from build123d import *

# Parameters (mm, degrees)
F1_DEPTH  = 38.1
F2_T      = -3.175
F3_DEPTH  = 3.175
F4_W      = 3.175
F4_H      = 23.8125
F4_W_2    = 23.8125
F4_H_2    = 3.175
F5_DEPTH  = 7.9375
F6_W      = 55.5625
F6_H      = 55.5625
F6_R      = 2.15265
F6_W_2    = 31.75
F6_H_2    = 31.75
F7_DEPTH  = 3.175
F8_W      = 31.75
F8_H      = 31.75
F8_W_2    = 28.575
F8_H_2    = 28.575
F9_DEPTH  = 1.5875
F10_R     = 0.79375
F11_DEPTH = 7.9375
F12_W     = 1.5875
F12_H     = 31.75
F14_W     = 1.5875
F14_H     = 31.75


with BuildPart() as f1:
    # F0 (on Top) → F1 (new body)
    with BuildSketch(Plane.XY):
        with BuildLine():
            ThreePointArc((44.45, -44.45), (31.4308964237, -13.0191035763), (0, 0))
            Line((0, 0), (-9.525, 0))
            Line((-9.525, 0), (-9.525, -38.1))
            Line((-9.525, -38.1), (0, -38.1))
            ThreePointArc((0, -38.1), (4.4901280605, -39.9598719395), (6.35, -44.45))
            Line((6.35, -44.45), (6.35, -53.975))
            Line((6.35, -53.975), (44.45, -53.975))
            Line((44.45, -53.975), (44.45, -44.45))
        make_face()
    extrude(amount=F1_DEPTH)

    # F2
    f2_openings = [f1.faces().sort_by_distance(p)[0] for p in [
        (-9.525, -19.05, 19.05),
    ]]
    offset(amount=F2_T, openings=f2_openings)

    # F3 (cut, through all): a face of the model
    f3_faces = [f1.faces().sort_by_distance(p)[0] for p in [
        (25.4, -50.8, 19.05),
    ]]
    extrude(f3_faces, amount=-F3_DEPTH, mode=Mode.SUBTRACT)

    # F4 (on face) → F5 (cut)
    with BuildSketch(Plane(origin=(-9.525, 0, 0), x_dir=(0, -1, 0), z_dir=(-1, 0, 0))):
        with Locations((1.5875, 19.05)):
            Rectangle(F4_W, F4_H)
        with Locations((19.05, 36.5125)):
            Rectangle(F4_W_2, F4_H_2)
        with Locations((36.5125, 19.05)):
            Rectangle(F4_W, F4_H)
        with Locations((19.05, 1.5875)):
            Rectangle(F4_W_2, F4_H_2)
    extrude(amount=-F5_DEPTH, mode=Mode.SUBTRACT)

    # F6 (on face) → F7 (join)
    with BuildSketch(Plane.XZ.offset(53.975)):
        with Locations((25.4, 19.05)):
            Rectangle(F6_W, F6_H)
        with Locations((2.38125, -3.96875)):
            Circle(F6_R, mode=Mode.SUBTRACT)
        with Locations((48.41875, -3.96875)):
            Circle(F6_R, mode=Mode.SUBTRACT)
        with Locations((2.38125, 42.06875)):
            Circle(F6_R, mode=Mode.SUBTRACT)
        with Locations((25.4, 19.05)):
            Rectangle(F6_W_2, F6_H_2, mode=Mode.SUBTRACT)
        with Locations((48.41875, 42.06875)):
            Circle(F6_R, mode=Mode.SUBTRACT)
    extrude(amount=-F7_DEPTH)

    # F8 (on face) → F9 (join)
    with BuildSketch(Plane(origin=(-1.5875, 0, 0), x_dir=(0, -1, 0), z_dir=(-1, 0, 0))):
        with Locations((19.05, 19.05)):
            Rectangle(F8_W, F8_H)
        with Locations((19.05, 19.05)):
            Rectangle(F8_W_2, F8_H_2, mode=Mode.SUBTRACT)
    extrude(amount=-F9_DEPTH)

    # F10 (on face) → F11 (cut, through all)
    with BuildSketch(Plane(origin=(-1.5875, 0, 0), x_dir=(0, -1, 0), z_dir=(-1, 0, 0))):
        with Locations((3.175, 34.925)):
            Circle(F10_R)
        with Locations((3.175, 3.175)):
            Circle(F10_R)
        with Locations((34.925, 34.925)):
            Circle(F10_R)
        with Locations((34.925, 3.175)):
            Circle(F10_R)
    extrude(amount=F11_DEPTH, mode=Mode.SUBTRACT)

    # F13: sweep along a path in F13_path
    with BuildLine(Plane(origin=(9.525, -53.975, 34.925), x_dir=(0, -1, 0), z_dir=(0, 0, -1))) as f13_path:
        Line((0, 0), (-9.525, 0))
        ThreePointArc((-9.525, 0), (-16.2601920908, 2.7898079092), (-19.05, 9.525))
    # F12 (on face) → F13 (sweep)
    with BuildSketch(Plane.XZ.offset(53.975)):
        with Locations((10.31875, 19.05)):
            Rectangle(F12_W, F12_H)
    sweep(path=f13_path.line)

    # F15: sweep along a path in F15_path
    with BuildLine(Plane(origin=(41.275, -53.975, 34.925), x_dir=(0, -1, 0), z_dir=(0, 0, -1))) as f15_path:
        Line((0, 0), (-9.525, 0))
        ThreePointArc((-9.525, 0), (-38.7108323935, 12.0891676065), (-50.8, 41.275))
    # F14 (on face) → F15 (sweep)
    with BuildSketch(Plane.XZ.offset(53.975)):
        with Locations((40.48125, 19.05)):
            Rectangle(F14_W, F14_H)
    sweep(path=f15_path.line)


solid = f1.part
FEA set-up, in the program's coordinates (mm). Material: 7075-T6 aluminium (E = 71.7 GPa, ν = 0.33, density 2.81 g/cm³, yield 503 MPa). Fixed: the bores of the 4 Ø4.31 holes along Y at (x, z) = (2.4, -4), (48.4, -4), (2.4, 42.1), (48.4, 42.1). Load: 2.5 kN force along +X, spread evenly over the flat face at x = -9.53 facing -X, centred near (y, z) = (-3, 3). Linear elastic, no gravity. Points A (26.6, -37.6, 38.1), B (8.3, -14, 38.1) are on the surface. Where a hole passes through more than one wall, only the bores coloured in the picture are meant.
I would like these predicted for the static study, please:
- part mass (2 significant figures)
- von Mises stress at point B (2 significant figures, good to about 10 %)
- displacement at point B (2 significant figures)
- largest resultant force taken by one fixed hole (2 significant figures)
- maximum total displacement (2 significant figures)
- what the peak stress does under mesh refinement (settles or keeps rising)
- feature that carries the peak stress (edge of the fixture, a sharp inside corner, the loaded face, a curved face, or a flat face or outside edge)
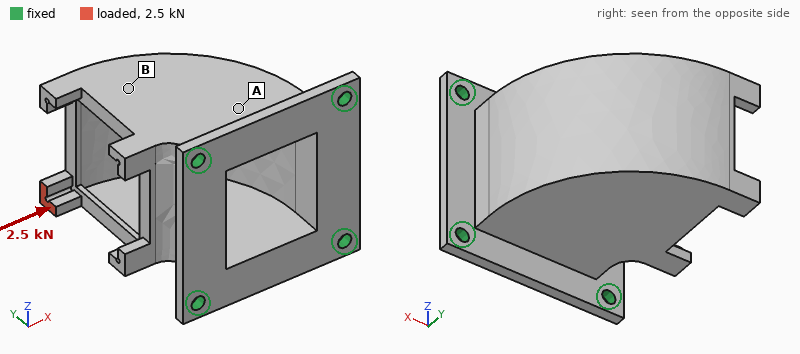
96 g
29 MPa
0.098 mm
2.2 kN
0.30 mm
keeps rising
edge of the fixture
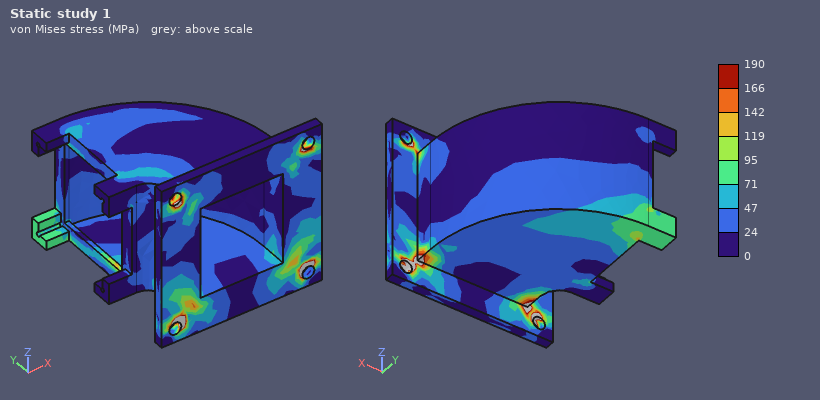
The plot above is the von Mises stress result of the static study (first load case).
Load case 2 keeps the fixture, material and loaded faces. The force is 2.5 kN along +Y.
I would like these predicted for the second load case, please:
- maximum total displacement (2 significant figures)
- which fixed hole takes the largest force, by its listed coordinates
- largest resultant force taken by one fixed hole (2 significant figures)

0.50 mm
(2.4, -4)
2.5 kN
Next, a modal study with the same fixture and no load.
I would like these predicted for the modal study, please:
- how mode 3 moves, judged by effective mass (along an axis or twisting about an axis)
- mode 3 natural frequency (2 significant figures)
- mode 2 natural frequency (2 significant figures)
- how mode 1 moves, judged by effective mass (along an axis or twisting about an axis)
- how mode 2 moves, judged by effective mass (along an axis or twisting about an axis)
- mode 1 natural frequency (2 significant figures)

along Y
6300 Hz
3600 Hz
along Z
along X
2900 Hz
